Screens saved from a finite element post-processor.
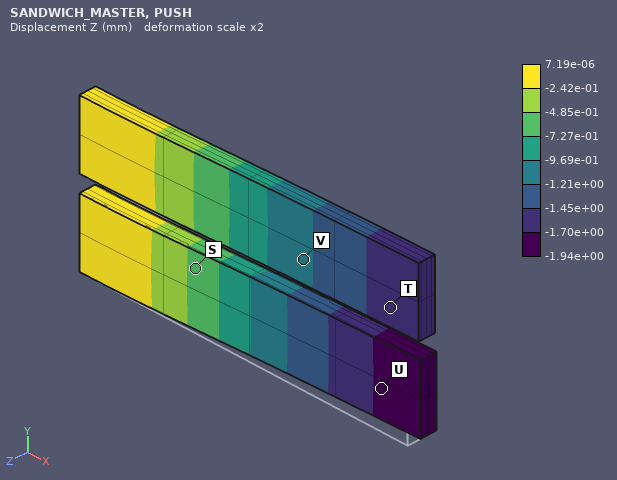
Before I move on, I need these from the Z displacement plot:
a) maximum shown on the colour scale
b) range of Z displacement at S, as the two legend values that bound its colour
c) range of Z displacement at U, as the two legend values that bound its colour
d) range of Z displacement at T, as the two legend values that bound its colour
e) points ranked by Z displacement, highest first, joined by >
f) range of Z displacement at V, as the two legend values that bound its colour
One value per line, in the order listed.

7.19e-06 mm
-7.27e-01 to -4.85e-01 mm
-1.94e+00 to -1.70e+00 mm
-1.70e+00 to -1.45e+00 mm
S > V > T > U
-1.21e+00 to -9.69e-01 mm
